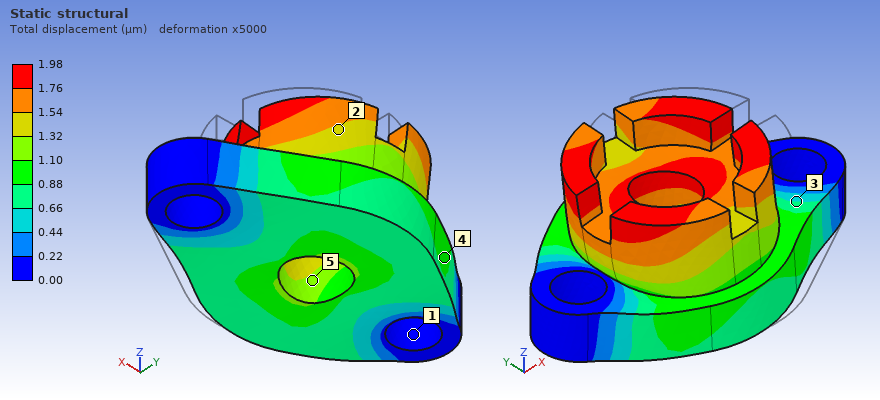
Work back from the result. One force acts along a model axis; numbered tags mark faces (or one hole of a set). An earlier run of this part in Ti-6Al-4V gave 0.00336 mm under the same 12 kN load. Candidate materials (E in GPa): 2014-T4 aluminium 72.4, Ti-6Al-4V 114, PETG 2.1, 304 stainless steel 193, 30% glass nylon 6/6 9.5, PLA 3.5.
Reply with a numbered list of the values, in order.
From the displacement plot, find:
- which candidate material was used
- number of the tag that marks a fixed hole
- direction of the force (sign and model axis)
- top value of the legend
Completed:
1. 304 stainless steel
2. 1
3. -X
4. 1.98 µm
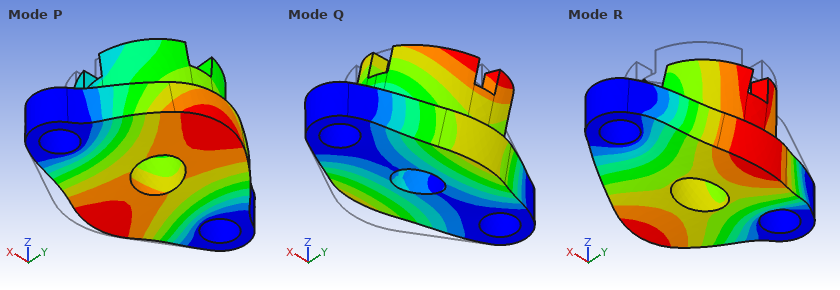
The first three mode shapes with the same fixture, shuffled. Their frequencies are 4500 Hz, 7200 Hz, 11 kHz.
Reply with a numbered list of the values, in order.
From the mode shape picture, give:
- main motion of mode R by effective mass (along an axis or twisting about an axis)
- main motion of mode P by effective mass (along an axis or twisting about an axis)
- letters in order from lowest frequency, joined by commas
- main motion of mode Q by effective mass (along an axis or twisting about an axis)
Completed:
1. along Z
2. along Y
3. Q, R, P
4. along Y
